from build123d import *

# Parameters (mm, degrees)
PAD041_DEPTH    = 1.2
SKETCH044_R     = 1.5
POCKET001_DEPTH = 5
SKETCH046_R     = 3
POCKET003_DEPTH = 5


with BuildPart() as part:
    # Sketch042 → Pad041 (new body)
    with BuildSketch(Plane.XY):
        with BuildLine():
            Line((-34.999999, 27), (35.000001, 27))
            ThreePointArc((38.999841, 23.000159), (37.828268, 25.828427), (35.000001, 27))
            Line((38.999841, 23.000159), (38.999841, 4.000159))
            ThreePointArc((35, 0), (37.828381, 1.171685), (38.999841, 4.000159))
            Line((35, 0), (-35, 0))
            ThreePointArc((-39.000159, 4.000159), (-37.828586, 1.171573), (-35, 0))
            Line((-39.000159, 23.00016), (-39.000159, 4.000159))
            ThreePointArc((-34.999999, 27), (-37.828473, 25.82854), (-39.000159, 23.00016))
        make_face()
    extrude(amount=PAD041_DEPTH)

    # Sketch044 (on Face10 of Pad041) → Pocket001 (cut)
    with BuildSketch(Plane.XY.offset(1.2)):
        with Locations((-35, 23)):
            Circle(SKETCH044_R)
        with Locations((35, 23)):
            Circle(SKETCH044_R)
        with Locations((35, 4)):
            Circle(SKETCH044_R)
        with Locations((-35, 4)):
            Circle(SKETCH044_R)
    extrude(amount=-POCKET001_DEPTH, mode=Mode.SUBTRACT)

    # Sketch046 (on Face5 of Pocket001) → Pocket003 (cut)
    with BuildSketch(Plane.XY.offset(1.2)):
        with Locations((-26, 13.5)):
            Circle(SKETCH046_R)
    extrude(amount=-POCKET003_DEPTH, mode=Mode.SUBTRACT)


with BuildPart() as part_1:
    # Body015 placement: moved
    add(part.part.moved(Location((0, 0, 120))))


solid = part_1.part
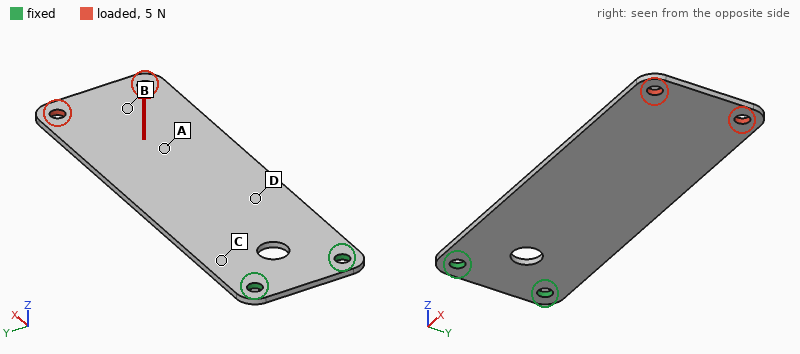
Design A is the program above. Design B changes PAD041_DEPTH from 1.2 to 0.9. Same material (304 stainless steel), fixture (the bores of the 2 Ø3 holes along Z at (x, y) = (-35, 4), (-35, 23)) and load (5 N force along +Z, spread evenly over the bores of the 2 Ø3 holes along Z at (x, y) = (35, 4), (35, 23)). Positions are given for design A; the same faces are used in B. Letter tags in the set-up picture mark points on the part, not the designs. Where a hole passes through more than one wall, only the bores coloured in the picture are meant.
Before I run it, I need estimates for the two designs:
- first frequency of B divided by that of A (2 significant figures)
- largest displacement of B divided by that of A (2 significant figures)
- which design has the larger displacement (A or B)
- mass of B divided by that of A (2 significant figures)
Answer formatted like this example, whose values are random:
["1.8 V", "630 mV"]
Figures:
["0.75", "2.4", "B", "0.75"]
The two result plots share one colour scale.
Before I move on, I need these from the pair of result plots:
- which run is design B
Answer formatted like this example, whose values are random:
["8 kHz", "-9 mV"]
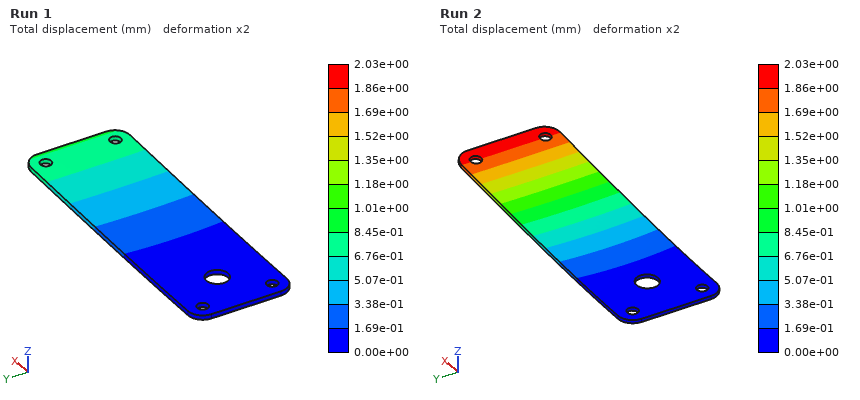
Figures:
["Run 2"]
